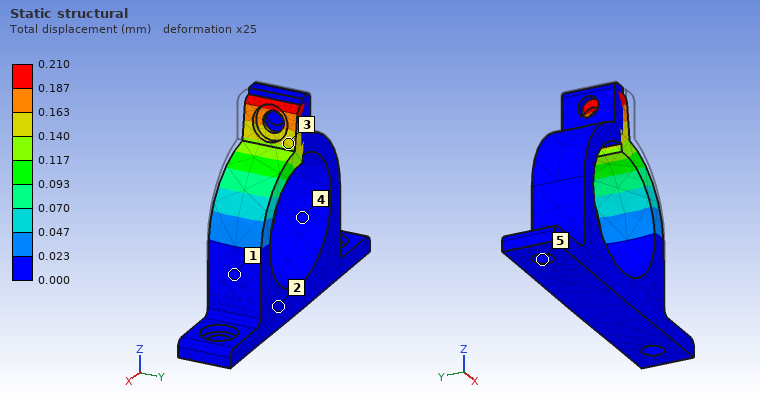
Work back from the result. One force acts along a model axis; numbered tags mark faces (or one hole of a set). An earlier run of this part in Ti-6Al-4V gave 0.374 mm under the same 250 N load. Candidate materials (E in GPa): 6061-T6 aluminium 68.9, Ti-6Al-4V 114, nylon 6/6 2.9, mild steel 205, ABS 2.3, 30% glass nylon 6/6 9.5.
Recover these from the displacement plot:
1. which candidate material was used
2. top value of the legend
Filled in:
mild steel
0.210 mm
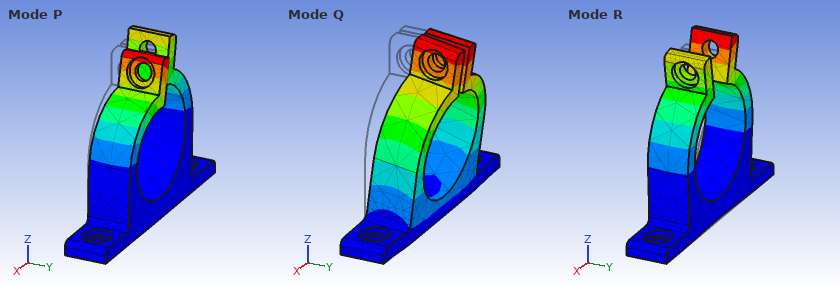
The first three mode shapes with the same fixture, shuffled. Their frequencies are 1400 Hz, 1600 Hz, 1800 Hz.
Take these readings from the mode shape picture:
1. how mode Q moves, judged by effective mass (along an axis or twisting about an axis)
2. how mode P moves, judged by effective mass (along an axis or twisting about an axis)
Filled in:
along Y
along X
